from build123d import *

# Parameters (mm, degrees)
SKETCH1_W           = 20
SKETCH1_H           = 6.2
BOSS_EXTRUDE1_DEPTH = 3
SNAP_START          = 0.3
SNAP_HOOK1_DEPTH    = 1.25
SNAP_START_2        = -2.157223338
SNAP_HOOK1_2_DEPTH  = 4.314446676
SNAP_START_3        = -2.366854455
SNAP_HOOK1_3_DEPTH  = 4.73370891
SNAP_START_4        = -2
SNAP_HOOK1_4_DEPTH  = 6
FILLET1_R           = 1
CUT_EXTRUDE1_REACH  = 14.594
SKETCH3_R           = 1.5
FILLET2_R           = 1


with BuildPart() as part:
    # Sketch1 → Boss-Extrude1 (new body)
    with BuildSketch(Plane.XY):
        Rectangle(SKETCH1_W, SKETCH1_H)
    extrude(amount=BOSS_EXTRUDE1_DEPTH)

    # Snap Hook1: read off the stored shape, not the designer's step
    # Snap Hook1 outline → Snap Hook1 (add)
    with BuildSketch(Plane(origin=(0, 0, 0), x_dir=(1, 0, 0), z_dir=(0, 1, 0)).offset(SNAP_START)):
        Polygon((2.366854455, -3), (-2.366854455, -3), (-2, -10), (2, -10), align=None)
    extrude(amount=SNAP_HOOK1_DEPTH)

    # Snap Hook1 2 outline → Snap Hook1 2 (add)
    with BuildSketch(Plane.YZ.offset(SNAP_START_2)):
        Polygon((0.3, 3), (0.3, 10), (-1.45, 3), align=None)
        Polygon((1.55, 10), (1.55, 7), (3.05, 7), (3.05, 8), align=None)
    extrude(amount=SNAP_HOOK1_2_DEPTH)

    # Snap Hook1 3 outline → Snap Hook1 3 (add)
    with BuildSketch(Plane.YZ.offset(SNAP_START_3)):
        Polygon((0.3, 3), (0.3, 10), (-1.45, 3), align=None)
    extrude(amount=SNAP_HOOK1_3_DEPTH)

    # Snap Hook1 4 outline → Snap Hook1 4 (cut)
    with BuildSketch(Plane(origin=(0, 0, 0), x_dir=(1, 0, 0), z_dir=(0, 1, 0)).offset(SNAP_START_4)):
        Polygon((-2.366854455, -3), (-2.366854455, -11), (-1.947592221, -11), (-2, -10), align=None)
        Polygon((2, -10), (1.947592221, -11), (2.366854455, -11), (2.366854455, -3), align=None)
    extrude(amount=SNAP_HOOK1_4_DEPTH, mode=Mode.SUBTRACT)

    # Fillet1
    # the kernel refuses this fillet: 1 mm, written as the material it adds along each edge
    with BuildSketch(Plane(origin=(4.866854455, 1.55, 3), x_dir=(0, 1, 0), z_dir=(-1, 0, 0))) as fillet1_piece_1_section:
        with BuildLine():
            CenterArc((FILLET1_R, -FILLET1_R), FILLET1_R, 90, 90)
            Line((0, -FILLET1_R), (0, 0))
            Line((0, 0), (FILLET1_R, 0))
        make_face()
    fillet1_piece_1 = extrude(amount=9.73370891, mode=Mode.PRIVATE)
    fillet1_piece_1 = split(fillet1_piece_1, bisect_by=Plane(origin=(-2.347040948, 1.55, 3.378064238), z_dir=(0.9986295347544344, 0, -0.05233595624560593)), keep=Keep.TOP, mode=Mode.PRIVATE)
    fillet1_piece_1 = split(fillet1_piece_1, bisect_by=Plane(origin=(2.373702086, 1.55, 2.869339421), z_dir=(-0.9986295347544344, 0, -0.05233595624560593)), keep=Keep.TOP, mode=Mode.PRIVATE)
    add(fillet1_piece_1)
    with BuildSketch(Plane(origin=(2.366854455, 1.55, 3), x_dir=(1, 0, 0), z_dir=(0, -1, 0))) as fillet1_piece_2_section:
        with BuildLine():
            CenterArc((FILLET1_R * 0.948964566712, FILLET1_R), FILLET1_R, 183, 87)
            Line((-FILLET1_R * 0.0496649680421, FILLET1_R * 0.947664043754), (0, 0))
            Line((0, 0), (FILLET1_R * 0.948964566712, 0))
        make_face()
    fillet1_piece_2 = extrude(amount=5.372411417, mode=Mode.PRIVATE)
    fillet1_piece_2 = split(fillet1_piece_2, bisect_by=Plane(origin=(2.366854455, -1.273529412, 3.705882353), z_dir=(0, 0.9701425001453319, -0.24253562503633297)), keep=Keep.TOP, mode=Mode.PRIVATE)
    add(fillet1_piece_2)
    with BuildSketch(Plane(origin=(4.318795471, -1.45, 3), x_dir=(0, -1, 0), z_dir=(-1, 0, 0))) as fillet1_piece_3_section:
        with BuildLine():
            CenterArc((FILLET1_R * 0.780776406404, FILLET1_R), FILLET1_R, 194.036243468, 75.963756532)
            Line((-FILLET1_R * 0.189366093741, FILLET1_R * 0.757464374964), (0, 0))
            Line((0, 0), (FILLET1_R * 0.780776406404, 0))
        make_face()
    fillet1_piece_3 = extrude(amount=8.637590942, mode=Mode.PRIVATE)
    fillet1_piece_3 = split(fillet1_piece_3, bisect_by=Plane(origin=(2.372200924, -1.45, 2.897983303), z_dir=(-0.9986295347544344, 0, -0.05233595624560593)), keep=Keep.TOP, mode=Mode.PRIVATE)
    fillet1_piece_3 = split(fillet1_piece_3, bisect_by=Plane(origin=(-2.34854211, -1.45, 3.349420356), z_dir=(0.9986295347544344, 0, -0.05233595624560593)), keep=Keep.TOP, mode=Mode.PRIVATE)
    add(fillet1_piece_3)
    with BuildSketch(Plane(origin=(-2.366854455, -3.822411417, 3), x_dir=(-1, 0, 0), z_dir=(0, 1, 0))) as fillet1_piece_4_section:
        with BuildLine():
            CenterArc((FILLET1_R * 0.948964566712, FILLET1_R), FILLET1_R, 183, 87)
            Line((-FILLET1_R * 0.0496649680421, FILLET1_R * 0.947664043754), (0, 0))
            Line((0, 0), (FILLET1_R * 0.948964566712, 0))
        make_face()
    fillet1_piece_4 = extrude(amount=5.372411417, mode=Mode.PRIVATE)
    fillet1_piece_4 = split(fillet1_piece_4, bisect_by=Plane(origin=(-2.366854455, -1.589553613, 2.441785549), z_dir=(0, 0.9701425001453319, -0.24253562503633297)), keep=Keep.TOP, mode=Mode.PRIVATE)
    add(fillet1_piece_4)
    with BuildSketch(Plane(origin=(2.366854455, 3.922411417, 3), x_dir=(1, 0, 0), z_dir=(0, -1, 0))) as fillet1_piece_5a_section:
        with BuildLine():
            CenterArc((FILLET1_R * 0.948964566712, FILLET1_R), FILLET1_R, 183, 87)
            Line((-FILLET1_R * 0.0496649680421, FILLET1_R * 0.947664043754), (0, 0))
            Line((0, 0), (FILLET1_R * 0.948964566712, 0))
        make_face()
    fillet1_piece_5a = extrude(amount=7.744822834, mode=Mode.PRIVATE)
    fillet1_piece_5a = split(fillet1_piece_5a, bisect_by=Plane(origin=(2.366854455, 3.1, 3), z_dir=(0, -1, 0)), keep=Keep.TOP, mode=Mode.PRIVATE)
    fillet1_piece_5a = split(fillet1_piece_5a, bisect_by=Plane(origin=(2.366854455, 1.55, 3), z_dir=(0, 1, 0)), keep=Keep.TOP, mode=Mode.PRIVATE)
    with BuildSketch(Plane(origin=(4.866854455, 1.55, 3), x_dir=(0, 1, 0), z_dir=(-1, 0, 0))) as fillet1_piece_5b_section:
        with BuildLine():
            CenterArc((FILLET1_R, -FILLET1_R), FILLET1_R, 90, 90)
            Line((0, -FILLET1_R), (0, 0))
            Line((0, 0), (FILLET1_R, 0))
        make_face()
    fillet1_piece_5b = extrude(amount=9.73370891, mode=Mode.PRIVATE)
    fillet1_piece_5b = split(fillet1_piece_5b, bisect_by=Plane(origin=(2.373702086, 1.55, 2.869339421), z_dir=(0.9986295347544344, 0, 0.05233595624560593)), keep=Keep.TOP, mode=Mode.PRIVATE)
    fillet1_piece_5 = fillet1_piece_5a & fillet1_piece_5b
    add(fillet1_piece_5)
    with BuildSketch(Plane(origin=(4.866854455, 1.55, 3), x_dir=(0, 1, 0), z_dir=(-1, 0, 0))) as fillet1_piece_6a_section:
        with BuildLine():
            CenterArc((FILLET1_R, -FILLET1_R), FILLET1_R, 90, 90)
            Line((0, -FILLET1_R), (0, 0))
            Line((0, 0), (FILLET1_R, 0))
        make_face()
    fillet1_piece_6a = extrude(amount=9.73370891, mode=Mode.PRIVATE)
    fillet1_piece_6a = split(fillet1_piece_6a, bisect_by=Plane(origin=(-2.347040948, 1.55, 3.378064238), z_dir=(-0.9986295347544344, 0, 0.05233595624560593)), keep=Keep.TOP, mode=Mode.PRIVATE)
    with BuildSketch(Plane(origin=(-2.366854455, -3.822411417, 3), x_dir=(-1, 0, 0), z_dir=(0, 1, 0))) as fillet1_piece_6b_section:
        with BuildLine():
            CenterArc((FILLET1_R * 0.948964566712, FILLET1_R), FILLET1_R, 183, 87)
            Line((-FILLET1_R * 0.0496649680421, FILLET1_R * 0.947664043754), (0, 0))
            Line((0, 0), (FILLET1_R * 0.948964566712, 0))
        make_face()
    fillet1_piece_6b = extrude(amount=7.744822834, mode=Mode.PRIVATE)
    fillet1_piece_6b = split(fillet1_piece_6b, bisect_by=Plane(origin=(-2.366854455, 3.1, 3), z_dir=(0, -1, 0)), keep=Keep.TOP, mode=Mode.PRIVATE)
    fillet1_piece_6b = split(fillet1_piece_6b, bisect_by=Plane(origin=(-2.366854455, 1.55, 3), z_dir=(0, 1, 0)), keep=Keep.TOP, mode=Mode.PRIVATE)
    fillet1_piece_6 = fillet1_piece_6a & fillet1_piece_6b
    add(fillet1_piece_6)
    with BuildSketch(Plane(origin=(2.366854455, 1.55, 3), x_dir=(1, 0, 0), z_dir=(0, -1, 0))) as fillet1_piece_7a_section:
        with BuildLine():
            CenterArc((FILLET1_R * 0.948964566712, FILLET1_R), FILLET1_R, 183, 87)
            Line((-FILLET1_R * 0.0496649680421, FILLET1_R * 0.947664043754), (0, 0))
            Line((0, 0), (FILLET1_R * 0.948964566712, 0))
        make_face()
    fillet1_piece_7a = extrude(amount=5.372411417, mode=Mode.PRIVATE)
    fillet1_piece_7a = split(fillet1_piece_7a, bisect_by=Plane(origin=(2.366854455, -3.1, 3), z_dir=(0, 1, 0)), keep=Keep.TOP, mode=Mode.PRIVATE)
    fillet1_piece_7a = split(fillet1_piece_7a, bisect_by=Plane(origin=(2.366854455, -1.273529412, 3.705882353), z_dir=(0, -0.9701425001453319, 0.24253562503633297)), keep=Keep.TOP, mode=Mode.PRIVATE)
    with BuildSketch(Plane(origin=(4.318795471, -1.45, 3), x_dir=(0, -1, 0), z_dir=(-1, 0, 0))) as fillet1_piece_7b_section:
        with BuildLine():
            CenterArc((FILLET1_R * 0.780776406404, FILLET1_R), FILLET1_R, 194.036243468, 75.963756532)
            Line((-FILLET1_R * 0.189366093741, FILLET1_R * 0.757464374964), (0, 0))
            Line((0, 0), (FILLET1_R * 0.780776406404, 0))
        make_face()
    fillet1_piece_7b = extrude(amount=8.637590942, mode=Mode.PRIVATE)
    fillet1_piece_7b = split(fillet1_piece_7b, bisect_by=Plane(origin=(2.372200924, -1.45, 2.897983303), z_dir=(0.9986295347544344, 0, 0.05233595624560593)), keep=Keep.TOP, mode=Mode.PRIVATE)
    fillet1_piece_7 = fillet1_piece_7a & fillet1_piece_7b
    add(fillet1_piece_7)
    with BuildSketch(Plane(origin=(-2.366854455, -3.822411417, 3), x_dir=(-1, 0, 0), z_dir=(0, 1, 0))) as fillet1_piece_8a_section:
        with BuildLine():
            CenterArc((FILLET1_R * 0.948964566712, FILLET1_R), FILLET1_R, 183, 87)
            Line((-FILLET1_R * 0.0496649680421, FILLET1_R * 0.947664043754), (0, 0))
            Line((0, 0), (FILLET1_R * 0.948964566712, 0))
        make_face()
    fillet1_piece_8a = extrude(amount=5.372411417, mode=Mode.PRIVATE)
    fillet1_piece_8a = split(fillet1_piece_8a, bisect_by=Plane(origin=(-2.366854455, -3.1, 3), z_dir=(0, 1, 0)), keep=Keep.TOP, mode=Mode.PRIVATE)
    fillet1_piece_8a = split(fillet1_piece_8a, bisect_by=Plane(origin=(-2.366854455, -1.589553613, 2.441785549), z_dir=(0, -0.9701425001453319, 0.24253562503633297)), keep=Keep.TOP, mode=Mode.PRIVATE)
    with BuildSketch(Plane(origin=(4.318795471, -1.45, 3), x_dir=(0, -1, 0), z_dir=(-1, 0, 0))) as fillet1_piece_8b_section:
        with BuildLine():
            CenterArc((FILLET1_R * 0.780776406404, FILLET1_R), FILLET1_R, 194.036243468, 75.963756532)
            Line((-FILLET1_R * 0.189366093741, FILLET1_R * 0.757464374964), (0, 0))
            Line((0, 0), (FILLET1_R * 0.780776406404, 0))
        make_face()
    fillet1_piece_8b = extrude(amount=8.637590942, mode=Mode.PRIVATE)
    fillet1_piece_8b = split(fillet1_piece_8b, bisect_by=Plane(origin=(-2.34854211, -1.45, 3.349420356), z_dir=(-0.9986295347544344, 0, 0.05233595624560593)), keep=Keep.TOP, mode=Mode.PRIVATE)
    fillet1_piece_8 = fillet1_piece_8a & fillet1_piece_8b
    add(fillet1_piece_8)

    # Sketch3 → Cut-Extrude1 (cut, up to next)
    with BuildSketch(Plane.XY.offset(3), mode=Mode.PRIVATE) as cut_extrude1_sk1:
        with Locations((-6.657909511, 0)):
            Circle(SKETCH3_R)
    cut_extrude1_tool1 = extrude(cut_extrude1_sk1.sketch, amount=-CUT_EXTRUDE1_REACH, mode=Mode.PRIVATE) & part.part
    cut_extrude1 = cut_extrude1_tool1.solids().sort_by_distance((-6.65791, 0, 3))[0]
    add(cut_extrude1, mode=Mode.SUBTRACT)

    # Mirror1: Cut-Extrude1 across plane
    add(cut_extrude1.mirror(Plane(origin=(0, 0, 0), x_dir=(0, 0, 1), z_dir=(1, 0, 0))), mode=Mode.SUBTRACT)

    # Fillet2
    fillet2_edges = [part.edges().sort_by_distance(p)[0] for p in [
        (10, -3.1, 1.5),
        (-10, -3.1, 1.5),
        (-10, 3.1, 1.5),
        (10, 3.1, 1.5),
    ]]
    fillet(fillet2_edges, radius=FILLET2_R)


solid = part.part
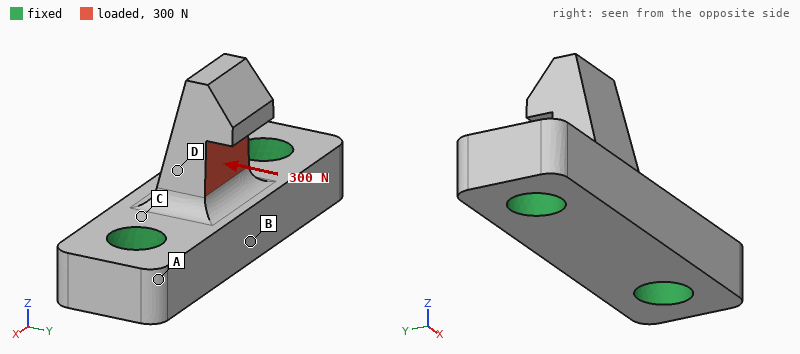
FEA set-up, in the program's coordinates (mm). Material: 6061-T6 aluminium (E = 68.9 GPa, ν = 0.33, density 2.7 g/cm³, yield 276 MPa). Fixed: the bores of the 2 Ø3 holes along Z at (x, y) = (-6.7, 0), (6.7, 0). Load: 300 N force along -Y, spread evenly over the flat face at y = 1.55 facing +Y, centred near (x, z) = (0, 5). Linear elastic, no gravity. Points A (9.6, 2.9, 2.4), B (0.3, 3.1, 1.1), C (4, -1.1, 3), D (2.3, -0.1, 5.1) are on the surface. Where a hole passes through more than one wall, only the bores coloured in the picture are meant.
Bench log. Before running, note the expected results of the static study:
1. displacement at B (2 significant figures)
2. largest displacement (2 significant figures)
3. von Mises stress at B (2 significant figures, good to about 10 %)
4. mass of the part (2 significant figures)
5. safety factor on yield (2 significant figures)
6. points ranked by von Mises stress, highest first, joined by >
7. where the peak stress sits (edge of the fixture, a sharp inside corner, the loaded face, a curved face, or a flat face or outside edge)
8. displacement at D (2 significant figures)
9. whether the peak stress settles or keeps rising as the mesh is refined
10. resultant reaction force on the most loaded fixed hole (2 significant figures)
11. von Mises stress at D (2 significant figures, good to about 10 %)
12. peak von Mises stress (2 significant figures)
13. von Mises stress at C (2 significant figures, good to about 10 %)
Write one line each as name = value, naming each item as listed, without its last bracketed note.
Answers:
displacement at B = 6.4 µm
largest displacement = 34 µm
von Mises stress at B = 27 MPa
mass of the part = 1.1 g
safety factor on yield = 1.4
points ranked by von Mises stress, highest first, joined by > = C > D > B > A
where the peak stress sits = a curved face
displacement at D = 13 µm
whether the peak stress settles or keeps rising as the mesh is refined = settles
resultant reaction force on the most loaded fixed hole = 150 N
von Mises stress at D = 48 MPa
peak von Mises stress = 200 MPa
von Mises stress at C = 67 MPa
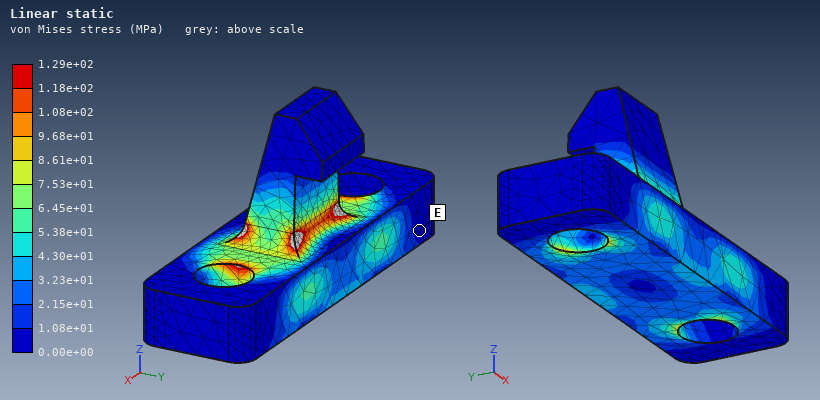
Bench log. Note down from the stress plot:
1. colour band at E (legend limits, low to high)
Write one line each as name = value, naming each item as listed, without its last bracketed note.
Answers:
colour band at E = 0.00e+00 to 1.08e+01 MPa
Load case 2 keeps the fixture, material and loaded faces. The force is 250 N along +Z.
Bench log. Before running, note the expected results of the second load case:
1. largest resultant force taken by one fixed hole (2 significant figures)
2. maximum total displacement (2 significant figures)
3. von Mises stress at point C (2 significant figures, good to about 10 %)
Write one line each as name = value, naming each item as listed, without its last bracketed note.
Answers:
largest resultant force taken by one fixed hole = 130 N
maximum total displacement = 17 µm
von Mises stress at point C = 14 MPa
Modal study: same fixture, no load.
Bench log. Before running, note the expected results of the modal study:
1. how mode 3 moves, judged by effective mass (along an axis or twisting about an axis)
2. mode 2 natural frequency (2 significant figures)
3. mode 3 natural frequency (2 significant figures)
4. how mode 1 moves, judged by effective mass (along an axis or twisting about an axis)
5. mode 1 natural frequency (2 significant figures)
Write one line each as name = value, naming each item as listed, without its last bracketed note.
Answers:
how mode 3 moves, judged by effective mass = along Z
mode 2 natural frequency = 53 kHz
mode 3 natural frequency = 71 kHz
how mode 1 moves, judged by effective mass = along Y
mode 1 natural frequency = 31 kHz
